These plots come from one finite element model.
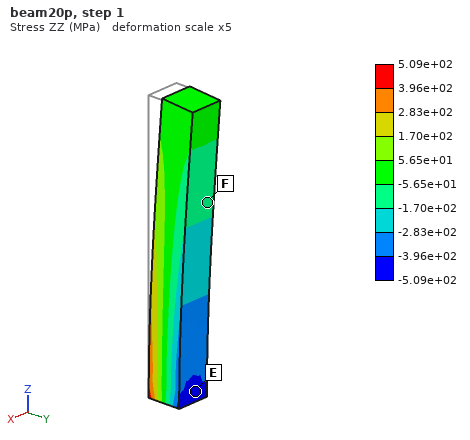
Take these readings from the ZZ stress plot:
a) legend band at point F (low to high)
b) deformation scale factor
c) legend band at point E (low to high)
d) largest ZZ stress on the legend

-1.70e+02 to -5.65e+01 MPa
5
-5.09e+02 to -3.96e+02 MPa
5.09e+02 MPa
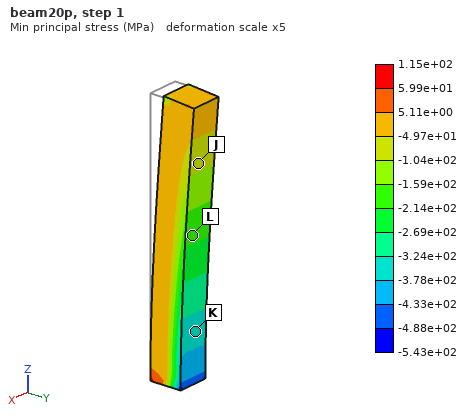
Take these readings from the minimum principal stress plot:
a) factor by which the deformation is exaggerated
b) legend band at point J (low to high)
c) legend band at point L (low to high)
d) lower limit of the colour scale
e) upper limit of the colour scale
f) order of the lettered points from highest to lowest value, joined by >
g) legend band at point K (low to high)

5
-1.04e+02 to -4.97e+01 MPa
-2.14e+02 to -1.59e+02 MPa
-5.43e+02 MPa
1.15e+02 MPa
J > L > K
-3.78e+02 to -3.24e+02 MPa
